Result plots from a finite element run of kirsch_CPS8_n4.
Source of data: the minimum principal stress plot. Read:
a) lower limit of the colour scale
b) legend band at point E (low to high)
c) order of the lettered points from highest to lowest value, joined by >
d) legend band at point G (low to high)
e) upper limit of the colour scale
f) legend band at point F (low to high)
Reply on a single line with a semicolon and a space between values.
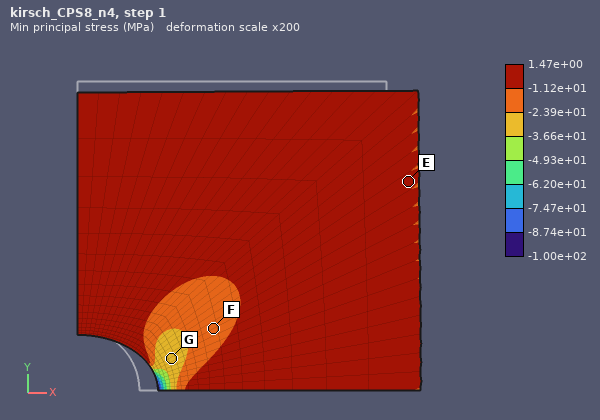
-1.00e+02 MPa; -1.12e+01 to 1.47e+00 MPa; E > F > G; -3.66e+01 to -2.39e+01 MPa; 1.47e+00 MPa; -2.39e+01 to -1.12e+01 MPa
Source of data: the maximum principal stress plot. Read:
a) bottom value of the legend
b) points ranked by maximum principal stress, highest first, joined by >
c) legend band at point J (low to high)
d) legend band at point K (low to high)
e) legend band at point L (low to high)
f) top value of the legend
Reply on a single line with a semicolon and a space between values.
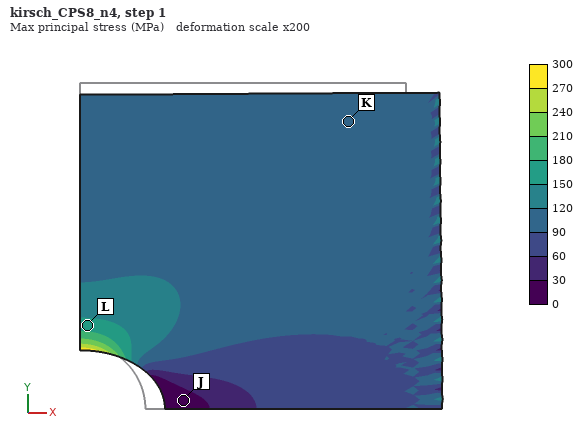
0 MPa; L > K > J; 0 to 30 MPa; 90 to 120 MPa; 150 to 180 MPa; 300 MPa
